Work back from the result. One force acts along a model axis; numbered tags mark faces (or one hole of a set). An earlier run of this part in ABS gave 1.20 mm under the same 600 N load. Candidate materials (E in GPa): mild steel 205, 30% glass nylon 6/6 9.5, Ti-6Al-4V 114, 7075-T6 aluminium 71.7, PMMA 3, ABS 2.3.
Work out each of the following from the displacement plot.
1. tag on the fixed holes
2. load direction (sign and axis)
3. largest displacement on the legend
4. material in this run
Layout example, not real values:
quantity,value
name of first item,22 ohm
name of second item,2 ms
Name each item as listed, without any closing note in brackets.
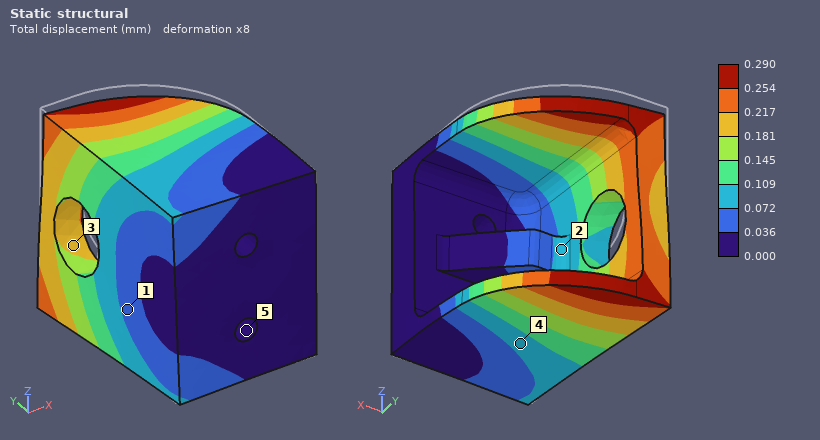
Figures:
quantity,value
tag on the fixed holes,5
load direction,-Z
largest displacement on the legend,0.290 mm
material in this run,30% glass nylon 6/6
